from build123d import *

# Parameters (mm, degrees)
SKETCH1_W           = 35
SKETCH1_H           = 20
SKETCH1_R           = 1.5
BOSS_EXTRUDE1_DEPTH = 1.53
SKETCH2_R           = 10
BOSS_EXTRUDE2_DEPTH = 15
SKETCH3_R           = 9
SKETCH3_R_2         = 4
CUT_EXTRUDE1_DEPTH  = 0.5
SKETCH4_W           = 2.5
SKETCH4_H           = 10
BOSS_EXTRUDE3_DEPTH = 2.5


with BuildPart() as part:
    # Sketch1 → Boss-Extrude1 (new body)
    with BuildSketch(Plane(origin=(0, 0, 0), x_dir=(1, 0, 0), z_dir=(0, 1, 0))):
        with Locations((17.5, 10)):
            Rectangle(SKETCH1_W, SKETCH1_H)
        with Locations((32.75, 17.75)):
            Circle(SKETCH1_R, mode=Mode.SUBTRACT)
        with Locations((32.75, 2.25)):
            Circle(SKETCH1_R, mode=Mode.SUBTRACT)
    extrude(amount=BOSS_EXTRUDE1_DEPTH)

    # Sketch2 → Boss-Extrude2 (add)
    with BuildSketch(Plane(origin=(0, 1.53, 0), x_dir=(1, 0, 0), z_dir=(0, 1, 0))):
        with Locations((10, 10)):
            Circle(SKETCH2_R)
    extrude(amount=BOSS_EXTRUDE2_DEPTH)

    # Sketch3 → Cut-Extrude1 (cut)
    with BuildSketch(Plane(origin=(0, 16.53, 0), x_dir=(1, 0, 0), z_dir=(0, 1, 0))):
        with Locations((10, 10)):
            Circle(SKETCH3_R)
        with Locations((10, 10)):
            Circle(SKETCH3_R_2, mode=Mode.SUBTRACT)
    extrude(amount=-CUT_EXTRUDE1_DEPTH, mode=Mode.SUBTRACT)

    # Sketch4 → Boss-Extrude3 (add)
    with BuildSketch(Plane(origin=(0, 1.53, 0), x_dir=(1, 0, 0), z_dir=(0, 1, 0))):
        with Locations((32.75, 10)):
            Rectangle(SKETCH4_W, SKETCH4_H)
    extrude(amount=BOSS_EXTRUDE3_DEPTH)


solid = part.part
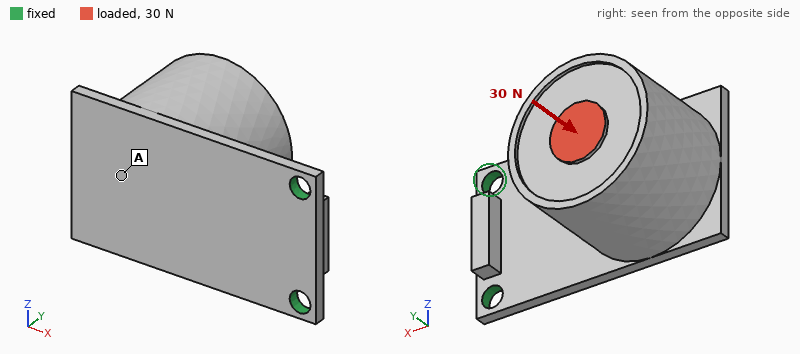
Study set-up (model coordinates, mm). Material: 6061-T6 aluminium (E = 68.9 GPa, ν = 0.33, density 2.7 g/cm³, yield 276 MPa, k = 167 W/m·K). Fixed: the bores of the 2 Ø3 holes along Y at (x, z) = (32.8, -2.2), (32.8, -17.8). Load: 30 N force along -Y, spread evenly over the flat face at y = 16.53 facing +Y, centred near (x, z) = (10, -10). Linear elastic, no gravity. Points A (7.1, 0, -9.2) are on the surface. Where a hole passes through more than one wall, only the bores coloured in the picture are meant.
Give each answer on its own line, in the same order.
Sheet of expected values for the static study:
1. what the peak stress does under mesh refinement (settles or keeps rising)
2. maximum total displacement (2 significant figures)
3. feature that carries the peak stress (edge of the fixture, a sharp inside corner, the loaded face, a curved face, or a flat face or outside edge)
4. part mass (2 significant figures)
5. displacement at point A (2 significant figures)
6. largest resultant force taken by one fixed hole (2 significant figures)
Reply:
keeps rising
0.45 mm
edge of the fixture
15 g
0.28 mm
15 N
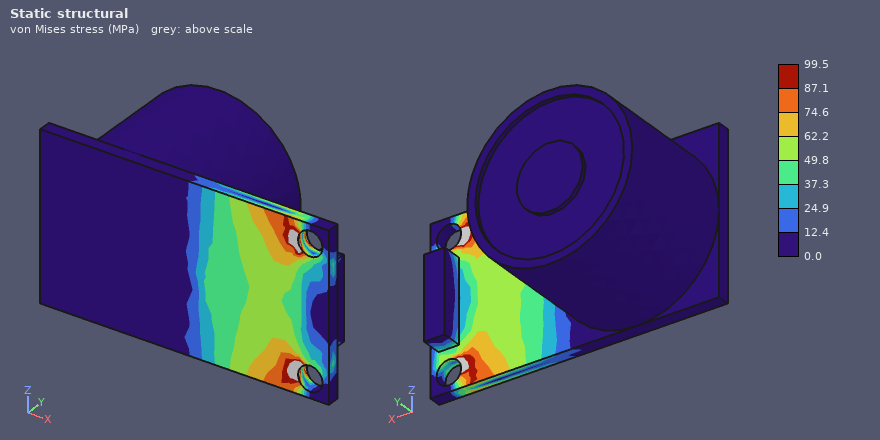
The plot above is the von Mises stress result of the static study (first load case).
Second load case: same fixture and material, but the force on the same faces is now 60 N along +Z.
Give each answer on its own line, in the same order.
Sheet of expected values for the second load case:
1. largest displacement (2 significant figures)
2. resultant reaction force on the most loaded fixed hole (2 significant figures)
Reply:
0.18 mm
110 N
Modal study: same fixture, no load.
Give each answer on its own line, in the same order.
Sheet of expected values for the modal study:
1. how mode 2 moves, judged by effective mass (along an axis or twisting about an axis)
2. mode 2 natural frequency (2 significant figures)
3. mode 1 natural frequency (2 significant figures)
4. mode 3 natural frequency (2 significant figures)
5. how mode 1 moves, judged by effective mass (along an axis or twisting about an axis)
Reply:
along Z
1300 Hz
400 Hz
3300 Hz
along Y
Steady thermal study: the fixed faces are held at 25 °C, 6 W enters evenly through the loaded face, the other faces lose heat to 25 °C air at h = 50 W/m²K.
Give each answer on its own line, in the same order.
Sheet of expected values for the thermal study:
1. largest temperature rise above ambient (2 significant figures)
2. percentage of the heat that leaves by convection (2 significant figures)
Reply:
18 K
26 %
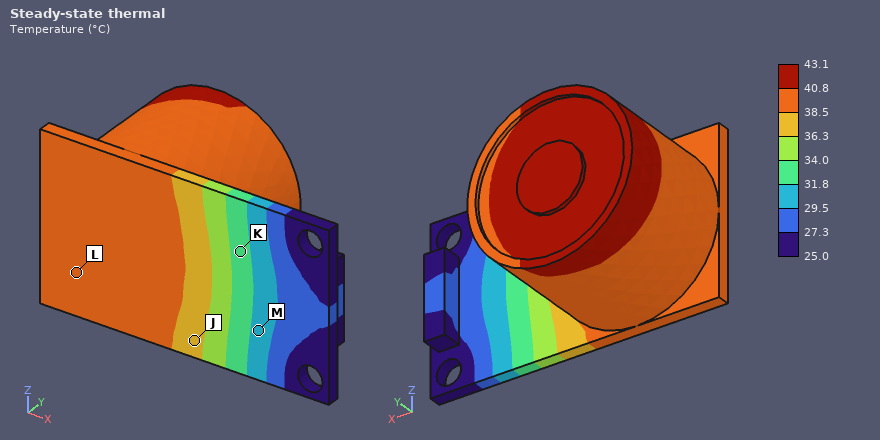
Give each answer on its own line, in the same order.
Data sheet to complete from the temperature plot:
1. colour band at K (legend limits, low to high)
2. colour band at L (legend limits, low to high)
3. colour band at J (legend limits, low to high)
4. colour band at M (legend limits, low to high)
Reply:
31.8 to 34.0 °C
38.5 to 40.8 °C
36.3 to 38.5 °C
29.5 to 31.8 °C
